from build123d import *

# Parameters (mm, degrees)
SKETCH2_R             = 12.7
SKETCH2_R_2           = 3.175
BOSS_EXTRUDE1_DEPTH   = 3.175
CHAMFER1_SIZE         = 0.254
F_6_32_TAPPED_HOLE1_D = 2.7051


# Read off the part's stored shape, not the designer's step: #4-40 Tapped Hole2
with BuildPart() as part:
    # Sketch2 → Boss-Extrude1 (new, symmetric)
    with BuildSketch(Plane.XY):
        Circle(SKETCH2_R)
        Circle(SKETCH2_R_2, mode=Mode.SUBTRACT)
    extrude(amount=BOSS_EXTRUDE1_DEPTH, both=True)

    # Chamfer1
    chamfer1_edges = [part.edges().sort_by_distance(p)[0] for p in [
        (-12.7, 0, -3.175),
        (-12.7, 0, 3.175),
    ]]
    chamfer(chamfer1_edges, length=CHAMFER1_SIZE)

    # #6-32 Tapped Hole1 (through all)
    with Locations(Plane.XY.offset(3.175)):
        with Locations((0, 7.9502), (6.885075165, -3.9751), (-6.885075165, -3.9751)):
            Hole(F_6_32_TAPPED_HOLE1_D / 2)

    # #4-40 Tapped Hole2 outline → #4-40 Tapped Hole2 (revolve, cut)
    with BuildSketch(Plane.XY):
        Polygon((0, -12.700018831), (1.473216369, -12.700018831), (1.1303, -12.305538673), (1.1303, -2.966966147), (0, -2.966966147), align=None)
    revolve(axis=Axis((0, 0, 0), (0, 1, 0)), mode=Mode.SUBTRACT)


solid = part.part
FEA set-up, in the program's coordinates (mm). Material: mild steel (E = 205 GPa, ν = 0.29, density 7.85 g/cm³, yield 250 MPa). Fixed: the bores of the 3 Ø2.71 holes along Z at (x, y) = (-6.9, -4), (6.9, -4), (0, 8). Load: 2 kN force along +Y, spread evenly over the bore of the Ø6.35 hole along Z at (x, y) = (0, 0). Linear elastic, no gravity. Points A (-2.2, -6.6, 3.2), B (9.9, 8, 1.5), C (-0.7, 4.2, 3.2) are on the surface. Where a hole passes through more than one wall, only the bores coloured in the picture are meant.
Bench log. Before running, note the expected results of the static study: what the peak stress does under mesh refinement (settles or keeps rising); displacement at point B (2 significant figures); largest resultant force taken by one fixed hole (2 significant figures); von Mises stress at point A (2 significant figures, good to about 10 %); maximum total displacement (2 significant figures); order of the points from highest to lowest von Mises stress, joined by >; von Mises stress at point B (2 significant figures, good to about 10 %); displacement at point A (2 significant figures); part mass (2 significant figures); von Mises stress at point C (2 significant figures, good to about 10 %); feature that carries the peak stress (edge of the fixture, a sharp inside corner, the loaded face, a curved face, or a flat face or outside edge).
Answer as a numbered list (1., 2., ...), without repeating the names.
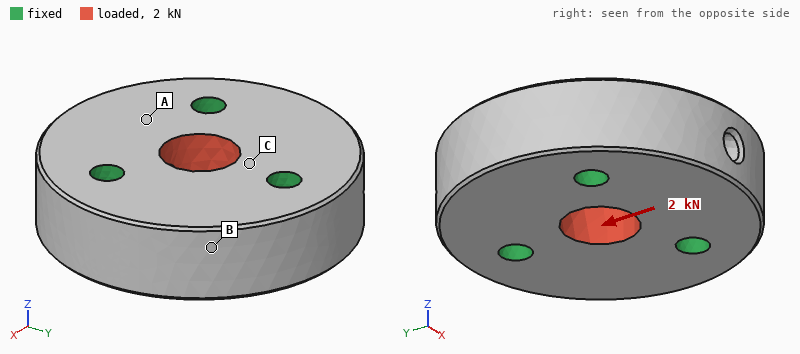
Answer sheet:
1. keeps rising
2. 0.20 µm
3. 680 N
4. 12 MPa
5. 0.73 µm
6. C > A > B
7. 4.0 MPa
8. 0.43 µm
9. 22 g
10. 21 MPa
11. edge of the fixture
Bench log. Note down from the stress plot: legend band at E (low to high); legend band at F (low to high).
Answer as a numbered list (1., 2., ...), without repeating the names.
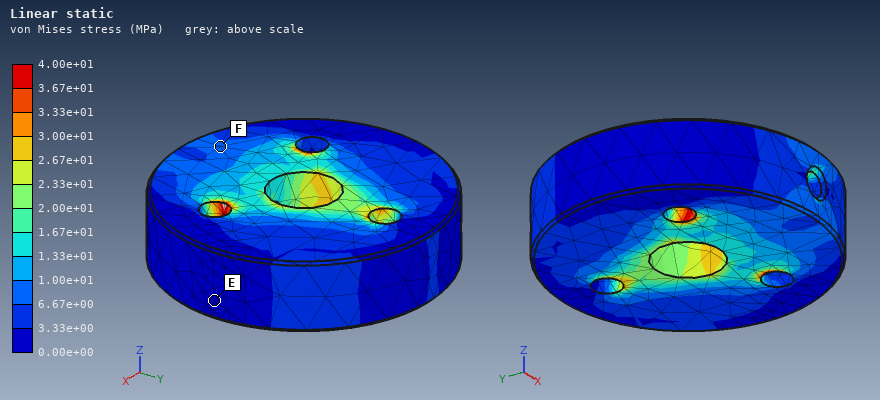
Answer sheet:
1. 0.00e+00 to 3.33e+00 MPa
2. 6.67e+00 to 1.00e+01 MPa
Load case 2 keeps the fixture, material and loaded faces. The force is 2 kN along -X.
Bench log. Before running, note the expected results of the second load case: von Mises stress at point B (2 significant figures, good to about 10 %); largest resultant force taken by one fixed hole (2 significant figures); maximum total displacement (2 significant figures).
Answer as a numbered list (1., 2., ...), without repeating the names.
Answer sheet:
1. 6.2 MPa
2. 700 N
3. 0.69 µm
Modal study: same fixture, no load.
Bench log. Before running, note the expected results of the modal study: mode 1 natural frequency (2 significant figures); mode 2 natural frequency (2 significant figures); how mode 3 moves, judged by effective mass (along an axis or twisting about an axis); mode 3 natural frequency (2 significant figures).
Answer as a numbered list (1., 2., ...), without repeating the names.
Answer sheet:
1. 53 kHz
2. 54 kHz
3. along Z
4. 60 kHz
